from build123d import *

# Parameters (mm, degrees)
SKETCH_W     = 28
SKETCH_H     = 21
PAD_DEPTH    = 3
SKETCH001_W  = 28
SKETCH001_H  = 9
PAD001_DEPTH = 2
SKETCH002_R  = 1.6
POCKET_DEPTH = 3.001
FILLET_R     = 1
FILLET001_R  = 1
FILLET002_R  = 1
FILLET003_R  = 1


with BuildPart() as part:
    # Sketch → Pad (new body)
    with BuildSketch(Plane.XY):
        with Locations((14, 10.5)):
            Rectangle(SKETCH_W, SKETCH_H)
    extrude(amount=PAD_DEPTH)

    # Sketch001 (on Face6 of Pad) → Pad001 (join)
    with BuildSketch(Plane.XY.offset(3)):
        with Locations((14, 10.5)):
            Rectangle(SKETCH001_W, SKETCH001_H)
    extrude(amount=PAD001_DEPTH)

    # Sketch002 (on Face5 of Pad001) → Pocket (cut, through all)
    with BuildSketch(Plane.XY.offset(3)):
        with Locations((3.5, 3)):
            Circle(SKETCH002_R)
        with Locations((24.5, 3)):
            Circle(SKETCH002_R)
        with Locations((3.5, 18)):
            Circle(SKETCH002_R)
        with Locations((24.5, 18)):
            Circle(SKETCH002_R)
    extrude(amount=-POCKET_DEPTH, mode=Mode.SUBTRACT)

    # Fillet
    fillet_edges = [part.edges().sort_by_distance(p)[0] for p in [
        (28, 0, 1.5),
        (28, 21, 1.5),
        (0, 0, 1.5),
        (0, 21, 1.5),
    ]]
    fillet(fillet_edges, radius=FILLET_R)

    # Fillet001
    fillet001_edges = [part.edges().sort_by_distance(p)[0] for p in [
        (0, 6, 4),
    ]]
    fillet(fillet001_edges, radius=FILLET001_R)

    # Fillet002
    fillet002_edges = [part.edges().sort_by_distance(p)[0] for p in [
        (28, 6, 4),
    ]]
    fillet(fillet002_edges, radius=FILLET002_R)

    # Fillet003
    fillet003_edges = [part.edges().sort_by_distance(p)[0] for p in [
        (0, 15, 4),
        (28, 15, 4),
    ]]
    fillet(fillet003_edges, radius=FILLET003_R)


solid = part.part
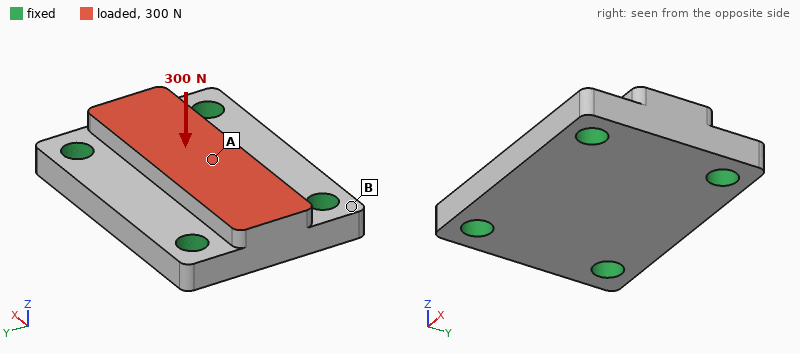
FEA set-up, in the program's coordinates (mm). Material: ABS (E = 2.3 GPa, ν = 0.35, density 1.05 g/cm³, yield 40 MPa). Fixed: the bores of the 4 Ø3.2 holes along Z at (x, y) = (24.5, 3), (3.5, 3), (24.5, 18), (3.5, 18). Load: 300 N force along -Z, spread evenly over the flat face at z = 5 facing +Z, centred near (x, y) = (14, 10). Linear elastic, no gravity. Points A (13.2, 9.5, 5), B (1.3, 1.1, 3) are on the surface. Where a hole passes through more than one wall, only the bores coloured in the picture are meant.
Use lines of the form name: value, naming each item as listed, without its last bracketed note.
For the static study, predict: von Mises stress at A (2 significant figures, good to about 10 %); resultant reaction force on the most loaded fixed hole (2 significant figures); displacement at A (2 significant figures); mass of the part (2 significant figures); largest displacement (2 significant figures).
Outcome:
von Mises stress at A: 3.9 MPa
resultant reaction force on the most loaded fixed hole: 81 N
displacement at A: 48 µm
mass of the part: 2.3 g
largest displacement: 48 µm
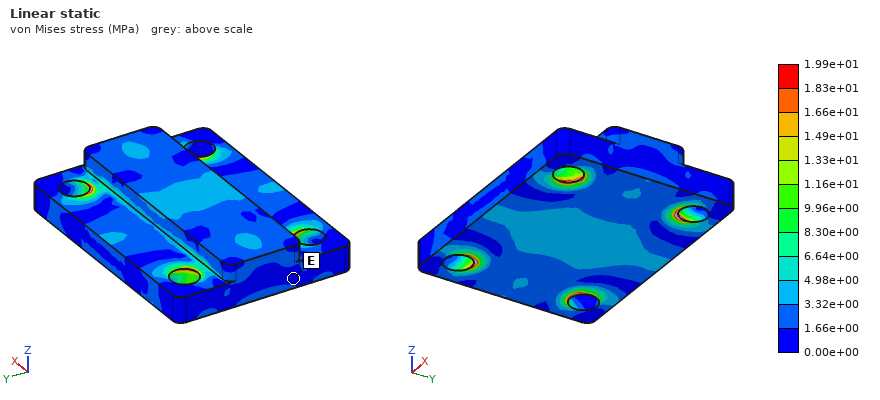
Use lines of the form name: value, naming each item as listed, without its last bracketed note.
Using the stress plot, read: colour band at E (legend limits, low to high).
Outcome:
colour band at E: 0.00e+00 to 1.66e+00 MPa
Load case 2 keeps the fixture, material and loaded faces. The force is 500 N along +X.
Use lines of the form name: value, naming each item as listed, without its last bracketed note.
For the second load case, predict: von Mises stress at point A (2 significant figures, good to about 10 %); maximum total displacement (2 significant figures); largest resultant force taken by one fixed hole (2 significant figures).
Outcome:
von Mises stress at point A: 3.5 MPa
maximum total displacement: 53 µm
largest resultant force taken by one fixed hole: 140 N
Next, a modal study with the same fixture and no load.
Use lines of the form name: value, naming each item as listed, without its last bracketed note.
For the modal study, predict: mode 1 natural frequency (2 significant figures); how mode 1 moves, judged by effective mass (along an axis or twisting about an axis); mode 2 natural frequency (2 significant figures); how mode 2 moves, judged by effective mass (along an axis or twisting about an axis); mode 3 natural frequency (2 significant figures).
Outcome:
mode 1 natural frequency: 9900 Hz
how mode 1 moves, judged by effective mass: along Z
mode 2 natural frequency: 13 kHz
how mode 2 moves, judged by effective mass: twisting about X
mode 3 natural frequency: 19 kHz
